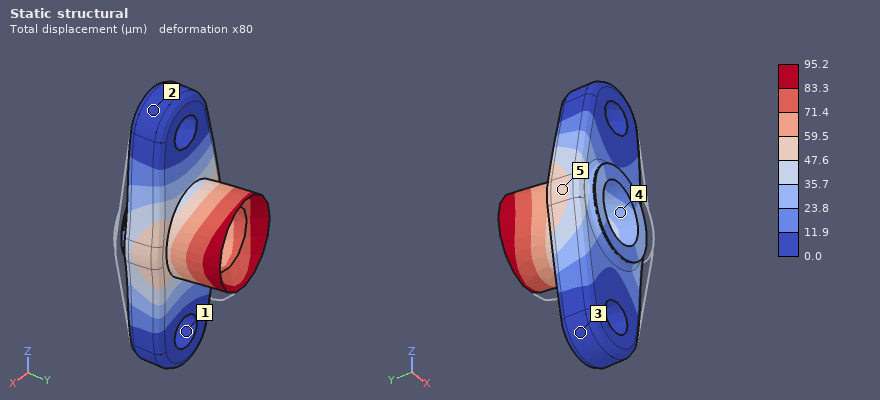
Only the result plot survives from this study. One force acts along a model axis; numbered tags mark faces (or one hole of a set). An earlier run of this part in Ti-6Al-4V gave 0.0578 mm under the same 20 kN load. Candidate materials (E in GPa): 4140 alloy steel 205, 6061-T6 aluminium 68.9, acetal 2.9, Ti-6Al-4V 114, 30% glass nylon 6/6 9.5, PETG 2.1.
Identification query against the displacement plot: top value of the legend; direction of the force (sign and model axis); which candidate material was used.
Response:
95.2 µm
-X
6061-T6 aluminium
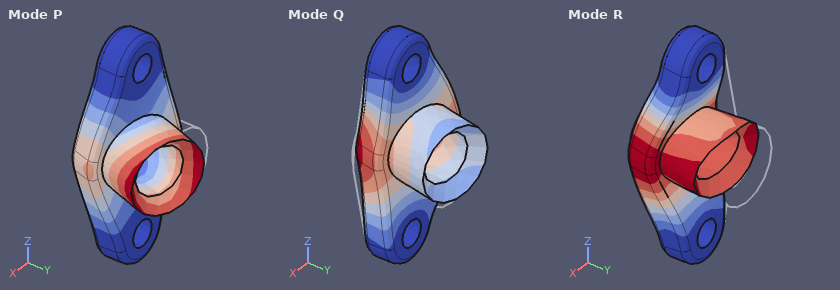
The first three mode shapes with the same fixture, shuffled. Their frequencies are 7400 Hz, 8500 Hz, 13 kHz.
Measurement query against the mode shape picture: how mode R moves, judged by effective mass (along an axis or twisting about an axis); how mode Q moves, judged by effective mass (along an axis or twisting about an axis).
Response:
along Y
along X
